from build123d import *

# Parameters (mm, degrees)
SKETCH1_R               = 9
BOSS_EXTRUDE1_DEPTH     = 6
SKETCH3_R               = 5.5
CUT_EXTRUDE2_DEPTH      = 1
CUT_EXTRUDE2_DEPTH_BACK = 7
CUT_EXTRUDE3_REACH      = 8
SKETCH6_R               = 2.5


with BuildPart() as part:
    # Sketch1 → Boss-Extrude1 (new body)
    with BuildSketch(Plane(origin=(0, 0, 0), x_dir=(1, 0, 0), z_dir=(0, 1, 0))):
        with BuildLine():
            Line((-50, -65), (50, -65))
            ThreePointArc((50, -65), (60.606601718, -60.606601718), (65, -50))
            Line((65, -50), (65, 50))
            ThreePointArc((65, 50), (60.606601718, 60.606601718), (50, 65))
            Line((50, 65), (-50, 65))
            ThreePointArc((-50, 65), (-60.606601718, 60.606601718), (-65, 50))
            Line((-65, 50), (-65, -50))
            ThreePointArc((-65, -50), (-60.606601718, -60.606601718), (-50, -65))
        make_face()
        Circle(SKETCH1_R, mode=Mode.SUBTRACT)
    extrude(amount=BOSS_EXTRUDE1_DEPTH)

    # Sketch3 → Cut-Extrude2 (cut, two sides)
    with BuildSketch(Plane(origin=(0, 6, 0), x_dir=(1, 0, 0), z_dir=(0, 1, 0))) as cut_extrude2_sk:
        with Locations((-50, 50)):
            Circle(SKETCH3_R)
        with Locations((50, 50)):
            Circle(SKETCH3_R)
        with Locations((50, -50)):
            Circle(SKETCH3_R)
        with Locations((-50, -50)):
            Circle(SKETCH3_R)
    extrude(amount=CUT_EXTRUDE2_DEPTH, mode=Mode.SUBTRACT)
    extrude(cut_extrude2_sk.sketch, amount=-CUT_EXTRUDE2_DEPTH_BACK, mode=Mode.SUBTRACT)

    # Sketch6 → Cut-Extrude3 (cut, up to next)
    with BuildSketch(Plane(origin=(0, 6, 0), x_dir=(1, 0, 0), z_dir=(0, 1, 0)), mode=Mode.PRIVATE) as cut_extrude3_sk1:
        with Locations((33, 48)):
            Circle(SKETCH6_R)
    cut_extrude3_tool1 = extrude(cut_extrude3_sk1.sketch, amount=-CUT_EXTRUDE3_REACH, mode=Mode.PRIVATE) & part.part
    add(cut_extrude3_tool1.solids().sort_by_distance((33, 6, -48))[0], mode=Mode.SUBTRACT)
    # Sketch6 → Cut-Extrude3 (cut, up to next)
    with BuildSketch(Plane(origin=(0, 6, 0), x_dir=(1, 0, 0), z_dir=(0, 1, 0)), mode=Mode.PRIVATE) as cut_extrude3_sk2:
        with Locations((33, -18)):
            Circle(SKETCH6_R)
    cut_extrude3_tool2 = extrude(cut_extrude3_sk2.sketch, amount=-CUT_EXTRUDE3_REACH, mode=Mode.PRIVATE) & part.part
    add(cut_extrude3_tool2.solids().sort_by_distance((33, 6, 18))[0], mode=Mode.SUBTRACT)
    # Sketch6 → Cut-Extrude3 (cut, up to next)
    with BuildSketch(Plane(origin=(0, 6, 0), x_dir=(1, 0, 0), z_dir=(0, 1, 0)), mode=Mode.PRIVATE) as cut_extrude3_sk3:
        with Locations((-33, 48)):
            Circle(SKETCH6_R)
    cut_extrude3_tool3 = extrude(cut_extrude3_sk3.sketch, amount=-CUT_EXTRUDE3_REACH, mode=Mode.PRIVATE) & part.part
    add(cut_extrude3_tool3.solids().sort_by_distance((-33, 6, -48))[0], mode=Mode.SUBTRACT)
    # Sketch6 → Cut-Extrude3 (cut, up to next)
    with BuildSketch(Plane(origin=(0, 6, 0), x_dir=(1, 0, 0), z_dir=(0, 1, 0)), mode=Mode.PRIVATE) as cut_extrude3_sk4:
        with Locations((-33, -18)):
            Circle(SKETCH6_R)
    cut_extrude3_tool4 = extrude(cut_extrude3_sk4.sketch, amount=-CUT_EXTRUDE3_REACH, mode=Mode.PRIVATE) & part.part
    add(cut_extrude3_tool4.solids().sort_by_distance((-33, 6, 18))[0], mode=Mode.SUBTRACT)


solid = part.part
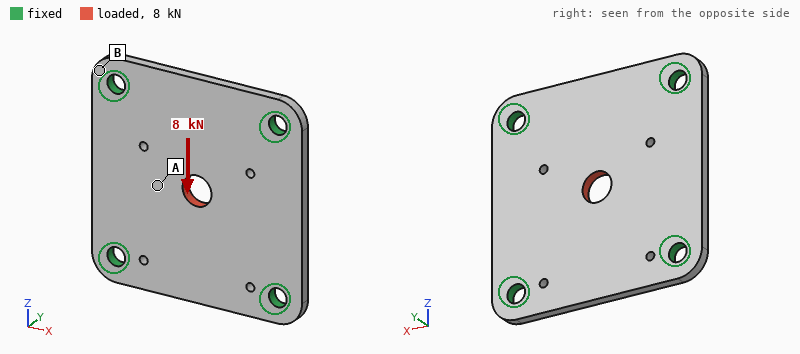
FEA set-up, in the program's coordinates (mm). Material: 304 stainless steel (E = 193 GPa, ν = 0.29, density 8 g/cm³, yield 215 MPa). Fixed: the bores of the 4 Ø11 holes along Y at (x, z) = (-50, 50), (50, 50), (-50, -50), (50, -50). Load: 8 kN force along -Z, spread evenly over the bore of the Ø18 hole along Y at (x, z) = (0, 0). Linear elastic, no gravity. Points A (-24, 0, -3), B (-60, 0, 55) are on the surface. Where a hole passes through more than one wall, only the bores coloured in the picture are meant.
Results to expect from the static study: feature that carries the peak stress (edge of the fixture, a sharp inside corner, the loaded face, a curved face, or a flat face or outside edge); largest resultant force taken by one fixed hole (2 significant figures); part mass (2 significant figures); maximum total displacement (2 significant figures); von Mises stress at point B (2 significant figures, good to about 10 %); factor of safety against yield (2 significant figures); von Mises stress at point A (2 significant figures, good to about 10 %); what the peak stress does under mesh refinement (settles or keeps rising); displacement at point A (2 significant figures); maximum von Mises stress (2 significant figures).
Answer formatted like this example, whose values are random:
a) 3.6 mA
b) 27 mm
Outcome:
a) the loaded face
b) 2.2 kN
c) 770 g
d) 5.5 µm
e) 4.6 MPa
f) 5.2
g) 10.0 MPa
h) settles
i) 2.9 µm
j) 41 MPa
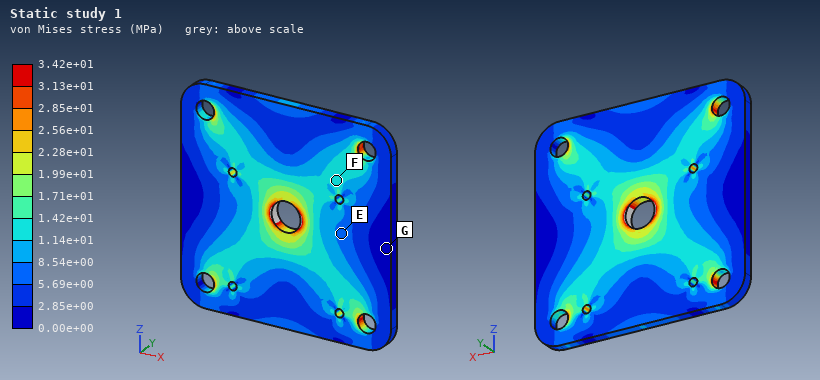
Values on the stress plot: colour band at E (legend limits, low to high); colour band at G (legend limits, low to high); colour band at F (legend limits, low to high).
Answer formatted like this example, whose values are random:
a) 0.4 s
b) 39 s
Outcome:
a) 5.69e+00 to 8.54e+00 MPa
b) 0.00e+00 to 2.85e+00 MPa
c) 1.14e+01 to 1.42e+01 MPa
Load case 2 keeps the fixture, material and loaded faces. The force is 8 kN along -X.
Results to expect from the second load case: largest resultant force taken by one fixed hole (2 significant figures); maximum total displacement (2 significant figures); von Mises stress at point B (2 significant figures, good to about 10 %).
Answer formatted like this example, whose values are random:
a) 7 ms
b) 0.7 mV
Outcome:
a) 2.2 kN
b) 5.5 µm
c) 5.3 MPa
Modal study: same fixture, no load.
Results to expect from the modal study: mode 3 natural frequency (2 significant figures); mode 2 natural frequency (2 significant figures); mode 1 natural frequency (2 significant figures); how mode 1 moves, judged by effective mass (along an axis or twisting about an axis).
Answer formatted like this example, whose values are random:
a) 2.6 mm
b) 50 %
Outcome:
a) 3600 Hz
b) 3600 Hz
c) 2300 Hz
d) along Y
